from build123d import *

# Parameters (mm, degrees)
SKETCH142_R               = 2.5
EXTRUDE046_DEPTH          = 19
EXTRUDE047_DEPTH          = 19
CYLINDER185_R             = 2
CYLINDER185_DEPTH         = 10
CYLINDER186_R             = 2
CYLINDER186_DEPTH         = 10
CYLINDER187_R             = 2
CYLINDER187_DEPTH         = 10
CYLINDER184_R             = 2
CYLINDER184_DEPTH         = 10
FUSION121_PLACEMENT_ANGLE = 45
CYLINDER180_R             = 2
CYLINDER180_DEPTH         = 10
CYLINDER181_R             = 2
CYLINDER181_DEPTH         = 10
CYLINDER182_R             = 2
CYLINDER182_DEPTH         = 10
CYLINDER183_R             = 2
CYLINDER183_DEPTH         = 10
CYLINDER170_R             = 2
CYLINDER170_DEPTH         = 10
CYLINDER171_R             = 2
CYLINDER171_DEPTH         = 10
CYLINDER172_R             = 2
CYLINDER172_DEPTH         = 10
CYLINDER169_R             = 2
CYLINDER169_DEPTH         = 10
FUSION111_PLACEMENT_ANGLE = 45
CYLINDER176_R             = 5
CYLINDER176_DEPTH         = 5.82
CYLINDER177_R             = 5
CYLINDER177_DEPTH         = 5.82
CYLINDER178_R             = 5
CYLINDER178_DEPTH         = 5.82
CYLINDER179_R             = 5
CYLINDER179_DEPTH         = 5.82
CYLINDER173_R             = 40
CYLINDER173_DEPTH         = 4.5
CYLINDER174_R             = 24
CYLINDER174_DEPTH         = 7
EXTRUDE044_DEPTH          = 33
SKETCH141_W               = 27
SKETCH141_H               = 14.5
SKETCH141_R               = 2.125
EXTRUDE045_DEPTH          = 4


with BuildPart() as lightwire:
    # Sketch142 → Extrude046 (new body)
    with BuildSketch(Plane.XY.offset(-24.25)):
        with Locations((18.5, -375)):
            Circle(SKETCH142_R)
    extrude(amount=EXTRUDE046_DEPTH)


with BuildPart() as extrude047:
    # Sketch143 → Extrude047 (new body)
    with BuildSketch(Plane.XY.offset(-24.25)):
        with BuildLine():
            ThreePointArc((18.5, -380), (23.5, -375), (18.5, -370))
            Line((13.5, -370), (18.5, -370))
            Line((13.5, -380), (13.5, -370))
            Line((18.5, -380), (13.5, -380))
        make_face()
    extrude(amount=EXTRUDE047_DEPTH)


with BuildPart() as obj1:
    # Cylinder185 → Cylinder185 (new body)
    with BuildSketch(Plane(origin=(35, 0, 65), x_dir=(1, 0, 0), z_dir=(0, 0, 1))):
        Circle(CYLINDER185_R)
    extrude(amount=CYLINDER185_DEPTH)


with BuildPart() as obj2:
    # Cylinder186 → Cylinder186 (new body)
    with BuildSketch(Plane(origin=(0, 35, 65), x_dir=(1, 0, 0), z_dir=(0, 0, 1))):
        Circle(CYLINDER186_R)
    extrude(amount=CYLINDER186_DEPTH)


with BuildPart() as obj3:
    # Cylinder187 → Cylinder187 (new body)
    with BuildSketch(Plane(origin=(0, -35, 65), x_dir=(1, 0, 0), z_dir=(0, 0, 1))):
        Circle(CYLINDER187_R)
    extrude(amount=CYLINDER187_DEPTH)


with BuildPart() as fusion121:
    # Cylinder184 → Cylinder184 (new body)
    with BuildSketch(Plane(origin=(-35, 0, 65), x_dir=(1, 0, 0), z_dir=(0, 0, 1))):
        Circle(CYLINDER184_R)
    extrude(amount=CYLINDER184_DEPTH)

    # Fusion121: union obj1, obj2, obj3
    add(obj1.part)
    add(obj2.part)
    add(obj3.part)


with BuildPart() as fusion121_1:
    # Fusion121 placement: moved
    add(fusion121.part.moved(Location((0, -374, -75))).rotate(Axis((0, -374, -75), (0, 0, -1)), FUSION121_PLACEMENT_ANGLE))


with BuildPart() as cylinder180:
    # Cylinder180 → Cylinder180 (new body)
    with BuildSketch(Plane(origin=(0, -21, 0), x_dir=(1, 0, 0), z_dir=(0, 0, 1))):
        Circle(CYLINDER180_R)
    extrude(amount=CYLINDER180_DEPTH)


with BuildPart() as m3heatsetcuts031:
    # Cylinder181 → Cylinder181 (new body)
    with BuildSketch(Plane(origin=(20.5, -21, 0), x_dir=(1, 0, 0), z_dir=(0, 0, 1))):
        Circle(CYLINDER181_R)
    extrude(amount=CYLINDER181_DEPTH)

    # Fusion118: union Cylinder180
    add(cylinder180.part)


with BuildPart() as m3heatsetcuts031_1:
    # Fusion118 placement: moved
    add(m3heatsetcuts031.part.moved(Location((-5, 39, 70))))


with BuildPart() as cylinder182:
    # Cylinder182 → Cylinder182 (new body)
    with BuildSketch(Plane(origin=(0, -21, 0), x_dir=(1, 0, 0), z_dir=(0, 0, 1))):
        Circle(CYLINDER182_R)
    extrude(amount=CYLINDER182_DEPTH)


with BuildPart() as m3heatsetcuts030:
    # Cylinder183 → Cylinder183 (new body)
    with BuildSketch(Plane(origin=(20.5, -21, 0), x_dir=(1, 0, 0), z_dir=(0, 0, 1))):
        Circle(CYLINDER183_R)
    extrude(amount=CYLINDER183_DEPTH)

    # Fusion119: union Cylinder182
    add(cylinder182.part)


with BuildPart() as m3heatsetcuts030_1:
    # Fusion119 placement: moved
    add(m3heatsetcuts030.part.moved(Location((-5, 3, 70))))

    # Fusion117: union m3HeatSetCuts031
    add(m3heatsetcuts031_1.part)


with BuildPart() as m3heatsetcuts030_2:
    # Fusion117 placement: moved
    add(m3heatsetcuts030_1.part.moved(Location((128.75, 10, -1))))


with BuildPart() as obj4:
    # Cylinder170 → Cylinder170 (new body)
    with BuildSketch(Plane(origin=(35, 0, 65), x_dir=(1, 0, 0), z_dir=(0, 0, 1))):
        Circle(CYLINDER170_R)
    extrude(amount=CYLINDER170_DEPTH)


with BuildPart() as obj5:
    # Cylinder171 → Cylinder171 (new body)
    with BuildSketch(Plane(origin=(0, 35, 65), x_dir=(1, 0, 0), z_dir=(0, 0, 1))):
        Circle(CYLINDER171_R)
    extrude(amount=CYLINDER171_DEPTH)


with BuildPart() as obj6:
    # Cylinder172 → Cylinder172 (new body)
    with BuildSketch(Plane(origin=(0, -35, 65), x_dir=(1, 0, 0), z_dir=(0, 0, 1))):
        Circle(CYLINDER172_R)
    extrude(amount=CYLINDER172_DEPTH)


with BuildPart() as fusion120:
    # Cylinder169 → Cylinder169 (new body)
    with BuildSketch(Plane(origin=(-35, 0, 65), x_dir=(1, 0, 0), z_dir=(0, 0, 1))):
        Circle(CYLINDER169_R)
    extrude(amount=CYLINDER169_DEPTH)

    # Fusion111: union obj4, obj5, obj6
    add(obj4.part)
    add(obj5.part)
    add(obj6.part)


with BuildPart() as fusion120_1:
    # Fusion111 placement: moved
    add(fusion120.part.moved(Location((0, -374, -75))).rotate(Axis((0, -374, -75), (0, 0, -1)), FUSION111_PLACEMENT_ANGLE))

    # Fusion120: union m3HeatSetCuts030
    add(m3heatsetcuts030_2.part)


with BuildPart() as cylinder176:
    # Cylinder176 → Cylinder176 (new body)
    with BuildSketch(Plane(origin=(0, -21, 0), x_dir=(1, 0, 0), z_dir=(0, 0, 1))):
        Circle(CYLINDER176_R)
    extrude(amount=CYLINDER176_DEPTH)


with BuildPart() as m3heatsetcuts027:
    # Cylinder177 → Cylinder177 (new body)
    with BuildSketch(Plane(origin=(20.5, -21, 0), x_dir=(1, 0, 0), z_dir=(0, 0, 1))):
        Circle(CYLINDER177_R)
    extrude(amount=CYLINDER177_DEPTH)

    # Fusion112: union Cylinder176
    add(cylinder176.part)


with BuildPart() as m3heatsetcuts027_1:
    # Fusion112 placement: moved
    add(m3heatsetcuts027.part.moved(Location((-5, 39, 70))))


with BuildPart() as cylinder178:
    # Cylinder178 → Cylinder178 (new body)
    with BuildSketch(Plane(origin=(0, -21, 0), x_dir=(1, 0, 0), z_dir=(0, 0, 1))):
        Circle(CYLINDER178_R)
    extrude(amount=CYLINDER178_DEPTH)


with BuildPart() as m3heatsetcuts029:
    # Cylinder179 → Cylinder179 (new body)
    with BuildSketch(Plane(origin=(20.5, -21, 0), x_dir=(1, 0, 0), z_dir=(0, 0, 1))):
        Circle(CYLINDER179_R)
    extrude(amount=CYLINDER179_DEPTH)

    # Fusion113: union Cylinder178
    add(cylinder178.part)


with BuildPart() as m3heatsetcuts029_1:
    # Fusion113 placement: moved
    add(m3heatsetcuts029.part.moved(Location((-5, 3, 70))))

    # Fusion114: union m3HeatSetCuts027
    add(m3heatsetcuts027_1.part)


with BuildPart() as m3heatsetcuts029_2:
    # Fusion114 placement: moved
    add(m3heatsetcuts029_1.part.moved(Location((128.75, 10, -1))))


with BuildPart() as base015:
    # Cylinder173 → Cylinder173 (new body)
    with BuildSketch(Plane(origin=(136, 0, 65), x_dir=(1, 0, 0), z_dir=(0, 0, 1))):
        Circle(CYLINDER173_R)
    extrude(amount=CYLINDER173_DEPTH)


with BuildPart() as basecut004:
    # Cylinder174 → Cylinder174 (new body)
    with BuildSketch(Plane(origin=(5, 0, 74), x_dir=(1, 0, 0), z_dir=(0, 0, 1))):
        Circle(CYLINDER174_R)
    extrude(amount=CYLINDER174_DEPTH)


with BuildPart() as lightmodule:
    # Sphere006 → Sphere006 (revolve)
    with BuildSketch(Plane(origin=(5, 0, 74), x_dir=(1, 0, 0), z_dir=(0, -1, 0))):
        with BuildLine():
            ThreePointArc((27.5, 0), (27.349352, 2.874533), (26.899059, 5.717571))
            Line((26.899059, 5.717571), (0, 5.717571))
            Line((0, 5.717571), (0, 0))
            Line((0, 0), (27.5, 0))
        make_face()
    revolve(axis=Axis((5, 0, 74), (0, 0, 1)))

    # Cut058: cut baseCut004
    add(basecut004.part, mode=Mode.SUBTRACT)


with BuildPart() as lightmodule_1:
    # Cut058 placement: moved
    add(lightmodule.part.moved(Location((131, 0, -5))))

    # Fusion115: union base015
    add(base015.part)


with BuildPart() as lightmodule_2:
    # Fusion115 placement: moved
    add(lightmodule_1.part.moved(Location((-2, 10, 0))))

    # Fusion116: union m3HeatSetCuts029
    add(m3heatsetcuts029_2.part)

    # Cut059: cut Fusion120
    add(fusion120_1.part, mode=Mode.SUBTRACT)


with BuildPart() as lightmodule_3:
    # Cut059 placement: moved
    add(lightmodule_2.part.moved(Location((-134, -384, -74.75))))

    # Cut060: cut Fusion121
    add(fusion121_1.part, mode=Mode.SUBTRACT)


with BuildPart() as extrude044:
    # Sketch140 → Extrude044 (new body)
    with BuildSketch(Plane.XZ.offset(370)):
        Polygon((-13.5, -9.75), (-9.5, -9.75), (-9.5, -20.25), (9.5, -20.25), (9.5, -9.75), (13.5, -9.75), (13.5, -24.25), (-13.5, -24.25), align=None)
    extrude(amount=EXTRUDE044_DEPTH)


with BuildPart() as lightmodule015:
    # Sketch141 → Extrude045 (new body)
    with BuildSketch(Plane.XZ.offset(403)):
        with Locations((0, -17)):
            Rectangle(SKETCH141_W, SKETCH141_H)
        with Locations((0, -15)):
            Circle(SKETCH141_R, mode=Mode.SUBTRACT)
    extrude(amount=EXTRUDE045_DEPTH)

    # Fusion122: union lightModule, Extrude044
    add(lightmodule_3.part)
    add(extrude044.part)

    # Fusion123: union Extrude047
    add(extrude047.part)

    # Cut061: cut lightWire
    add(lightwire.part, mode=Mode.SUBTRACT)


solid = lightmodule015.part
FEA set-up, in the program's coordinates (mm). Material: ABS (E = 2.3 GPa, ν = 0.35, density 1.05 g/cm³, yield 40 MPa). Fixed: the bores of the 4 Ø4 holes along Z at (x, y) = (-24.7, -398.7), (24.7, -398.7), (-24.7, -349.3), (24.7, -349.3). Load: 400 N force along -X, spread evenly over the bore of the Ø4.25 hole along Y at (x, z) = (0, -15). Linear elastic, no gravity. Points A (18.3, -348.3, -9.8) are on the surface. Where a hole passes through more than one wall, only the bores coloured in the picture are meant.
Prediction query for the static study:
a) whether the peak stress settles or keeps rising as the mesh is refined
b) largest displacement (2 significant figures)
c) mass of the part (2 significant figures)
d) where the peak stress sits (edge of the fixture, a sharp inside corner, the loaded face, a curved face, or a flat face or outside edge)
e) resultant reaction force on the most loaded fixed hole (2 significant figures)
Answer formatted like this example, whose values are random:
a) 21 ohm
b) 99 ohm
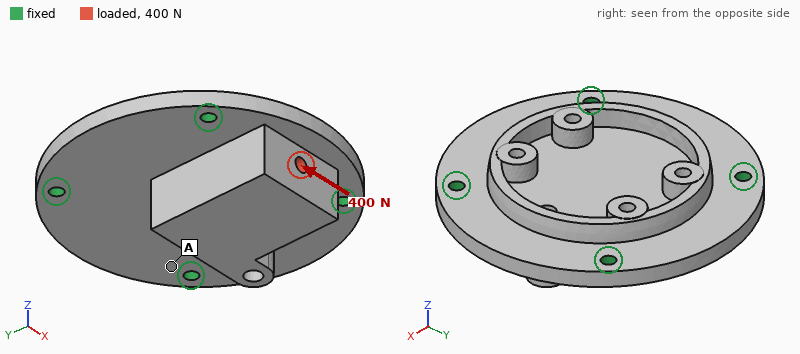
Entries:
a) keeps rising
b) 79 µm
c) 37 g
d) edge of the fixture
e) 200 N
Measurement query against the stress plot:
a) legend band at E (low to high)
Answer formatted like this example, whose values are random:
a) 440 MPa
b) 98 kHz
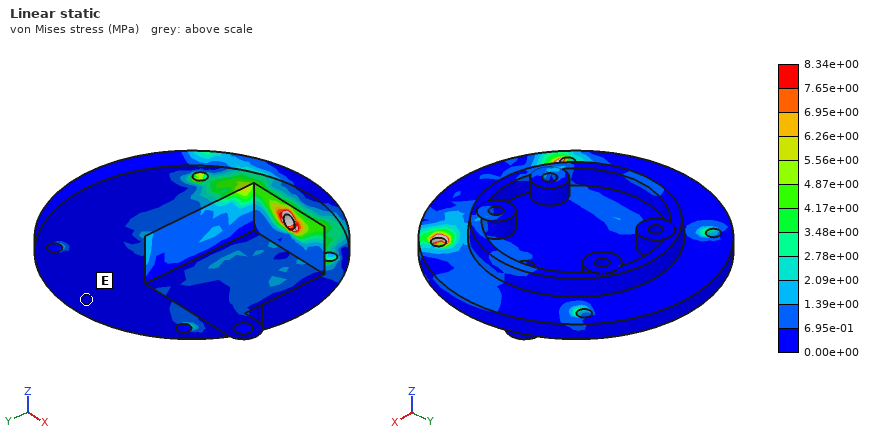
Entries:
a) 0.00e+00 to 6.95e-01 MPa
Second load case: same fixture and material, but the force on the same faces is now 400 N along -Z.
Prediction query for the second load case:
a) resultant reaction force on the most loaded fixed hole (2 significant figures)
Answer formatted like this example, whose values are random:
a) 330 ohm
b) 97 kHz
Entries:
a) 230 N
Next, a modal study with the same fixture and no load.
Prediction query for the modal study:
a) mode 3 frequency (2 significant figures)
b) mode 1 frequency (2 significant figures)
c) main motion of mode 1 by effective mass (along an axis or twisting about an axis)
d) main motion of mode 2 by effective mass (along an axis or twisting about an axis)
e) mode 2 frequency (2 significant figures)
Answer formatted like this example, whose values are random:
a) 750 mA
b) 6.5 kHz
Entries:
a) 2500 Hz
b) 1900 Hz
c) along Z
d) along Z
e) 2300 Hz
